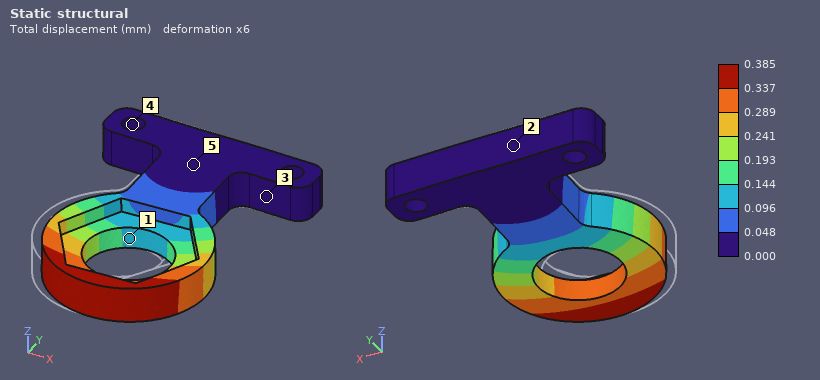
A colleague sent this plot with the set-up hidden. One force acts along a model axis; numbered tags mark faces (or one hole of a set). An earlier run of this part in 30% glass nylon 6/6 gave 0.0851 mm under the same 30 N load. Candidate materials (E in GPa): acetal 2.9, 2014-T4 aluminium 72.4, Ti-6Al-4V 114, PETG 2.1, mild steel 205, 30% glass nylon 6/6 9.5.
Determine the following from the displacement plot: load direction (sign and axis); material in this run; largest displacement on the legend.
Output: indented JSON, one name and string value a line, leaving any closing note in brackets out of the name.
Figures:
{
  "load direction": "+X",
  "material in this run": "PETG",
  "largest displacement on the legend": "0.385 mm"
}
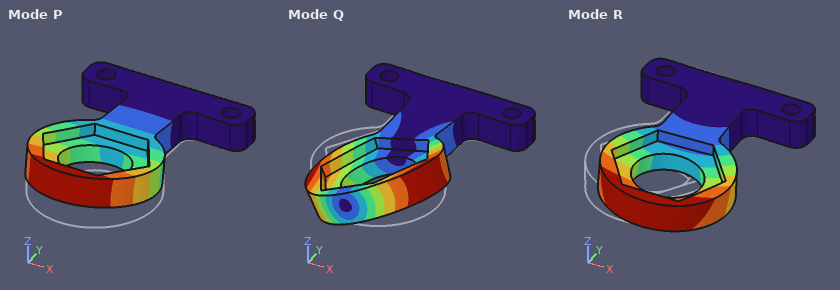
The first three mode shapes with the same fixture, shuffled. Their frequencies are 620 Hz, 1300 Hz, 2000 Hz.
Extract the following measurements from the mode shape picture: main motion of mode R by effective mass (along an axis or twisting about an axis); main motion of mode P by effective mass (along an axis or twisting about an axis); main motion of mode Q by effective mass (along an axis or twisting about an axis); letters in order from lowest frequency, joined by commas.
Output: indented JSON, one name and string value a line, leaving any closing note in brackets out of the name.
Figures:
{
  "main motion of mode R by effective mass": "along X",
  "main motion of mode P by effective mass": "along Z",
  "main motion of mode Q by effective mass": "twisting about Y",
  "letters in order from lowest frequency, joined by commas": "P, R, Q"
}
